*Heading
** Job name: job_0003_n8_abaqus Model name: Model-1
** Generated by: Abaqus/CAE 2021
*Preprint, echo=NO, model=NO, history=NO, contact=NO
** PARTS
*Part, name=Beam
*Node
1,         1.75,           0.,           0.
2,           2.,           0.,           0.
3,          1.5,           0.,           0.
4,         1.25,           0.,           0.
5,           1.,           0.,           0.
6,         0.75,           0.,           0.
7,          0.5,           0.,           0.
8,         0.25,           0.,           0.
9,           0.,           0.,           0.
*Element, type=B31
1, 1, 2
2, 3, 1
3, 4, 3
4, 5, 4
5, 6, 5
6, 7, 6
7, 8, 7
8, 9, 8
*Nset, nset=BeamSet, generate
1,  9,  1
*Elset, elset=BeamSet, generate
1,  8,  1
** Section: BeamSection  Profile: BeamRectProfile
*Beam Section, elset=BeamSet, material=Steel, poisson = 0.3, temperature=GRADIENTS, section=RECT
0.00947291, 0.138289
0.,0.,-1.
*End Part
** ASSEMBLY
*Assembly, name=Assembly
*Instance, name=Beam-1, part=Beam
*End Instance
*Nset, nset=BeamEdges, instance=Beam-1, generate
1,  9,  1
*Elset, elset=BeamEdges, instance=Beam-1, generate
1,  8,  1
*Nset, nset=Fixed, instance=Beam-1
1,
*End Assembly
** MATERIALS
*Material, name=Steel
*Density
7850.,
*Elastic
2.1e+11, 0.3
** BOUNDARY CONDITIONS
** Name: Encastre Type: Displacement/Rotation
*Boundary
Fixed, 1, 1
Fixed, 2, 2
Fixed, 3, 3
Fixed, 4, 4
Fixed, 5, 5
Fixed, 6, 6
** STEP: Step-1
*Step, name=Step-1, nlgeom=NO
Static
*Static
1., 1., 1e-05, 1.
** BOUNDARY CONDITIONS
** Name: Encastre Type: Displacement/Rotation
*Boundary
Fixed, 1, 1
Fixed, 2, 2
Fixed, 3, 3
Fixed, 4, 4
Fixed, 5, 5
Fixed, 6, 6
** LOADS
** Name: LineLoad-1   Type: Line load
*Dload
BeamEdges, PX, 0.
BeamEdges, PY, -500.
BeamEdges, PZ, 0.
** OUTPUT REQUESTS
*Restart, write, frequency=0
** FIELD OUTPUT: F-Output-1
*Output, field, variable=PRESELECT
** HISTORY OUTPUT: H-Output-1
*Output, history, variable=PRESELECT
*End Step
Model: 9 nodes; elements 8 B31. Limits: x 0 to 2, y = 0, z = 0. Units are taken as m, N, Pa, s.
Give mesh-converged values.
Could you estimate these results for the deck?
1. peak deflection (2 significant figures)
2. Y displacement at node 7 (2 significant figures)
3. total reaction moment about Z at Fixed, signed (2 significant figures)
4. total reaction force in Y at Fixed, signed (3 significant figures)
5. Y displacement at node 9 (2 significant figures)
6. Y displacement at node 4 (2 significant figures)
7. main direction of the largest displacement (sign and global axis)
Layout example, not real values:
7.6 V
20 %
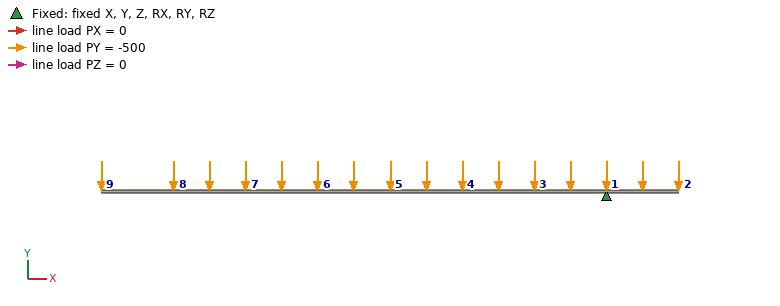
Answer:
0.0013 m
-8.4e-04 m
-750 N·m
1000 N
-0.0013 m
-1.8e-04 m
-Y
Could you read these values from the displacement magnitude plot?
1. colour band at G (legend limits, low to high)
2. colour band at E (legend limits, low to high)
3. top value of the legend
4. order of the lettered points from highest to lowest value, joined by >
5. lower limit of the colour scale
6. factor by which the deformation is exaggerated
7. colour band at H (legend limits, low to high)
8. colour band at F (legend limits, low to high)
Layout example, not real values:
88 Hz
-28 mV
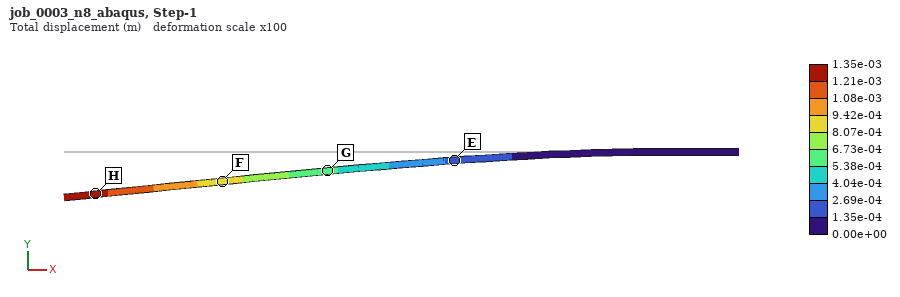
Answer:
5.38e-04 to 6.73e-04 m
1.35e-04 to 2.69e-04 m
1.35e-03 m
H > F > G > E
0.00e+00 m
100
1.21e-03 to 1.35e-03 m
8.07e-04 to 9.42e-04 m
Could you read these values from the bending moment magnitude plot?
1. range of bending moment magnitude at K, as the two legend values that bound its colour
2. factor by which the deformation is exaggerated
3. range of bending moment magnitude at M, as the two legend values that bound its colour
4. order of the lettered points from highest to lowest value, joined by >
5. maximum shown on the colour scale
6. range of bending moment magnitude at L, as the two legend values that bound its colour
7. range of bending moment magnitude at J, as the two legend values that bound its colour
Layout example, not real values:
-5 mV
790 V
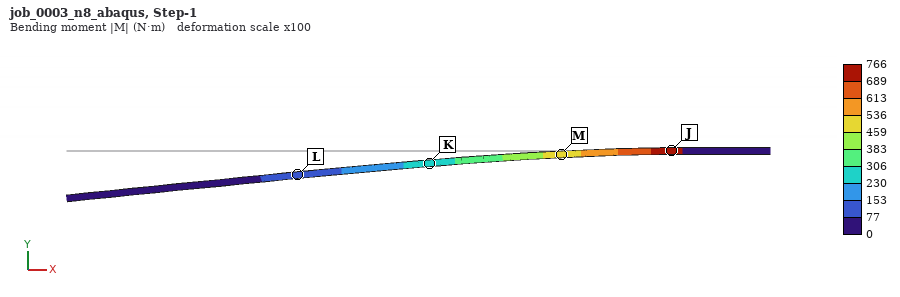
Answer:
230 to 306 N·m
100
459 to 536 N·m
J > M > K > L
766 N·m
77 to 153 N·m
689 to 766 N·m
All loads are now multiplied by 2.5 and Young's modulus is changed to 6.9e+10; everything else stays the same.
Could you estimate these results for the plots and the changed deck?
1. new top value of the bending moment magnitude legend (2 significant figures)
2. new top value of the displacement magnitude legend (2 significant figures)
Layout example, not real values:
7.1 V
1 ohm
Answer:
1900 N·m
0.010 m
